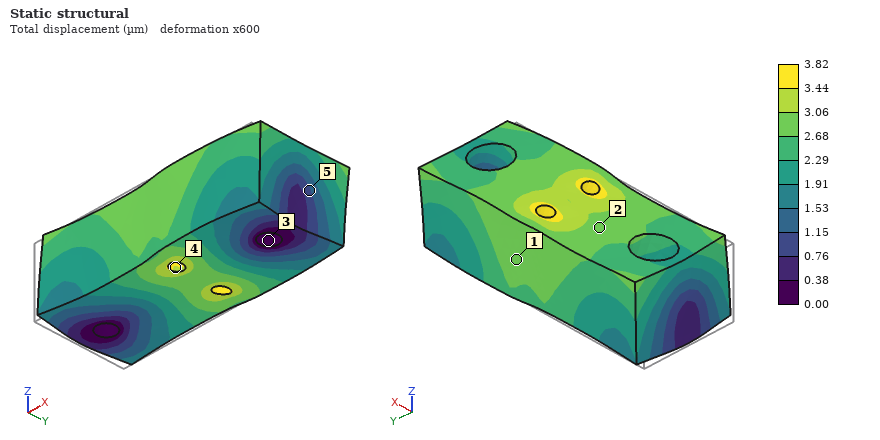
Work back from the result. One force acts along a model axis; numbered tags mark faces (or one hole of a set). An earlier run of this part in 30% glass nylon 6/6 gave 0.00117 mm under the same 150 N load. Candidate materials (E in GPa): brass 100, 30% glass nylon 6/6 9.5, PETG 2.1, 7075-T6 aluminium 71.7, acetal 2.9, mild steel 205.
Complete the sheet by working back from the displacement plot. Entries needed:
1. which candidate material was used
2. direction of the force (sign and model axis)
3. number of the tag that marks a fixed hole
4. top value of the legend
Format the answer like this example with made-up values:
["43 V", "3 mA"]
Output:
["acetal", "+X", "3", "3.82 µm"]
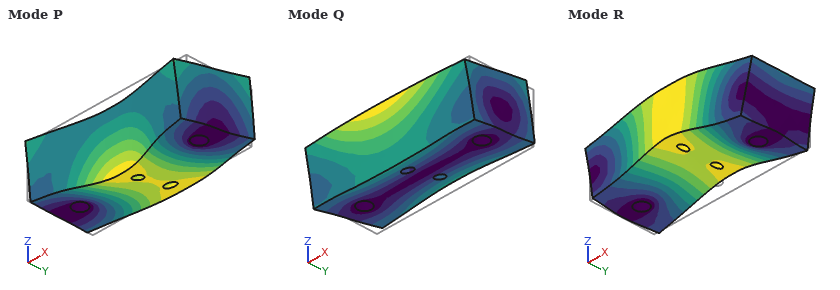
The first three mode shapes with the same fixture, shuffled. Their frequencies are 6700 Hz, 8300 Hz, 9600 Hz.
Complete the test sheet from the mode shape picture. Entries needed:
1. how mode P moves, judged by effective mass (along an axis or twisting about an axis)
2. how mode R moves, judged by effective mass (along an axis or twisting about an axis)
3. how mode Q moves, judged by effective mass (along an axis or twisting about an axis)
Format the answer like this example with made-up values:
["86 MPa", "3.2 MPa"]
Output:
["along Y", "along Z", "along Y"]
